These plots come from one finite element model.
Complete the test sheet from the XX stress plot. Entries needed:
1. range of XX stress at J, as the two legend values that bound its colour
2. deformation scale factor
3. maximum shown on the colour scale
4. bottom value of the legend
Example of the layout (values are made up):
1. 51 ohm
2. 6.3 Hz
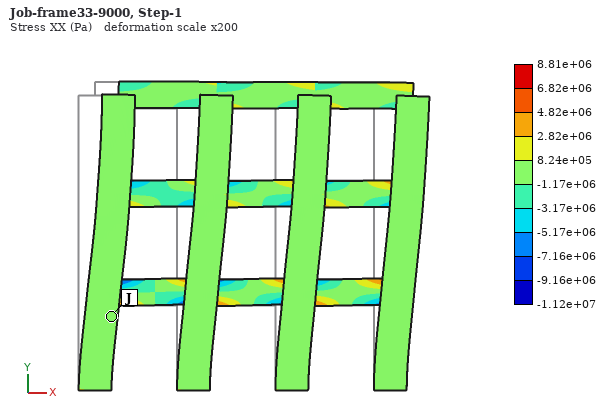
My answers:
1. -1.17e+06 to 8.24e+05 Pa
2. 200
3. 8.81e+06 Pa
4. -1.12e+07 Pa
